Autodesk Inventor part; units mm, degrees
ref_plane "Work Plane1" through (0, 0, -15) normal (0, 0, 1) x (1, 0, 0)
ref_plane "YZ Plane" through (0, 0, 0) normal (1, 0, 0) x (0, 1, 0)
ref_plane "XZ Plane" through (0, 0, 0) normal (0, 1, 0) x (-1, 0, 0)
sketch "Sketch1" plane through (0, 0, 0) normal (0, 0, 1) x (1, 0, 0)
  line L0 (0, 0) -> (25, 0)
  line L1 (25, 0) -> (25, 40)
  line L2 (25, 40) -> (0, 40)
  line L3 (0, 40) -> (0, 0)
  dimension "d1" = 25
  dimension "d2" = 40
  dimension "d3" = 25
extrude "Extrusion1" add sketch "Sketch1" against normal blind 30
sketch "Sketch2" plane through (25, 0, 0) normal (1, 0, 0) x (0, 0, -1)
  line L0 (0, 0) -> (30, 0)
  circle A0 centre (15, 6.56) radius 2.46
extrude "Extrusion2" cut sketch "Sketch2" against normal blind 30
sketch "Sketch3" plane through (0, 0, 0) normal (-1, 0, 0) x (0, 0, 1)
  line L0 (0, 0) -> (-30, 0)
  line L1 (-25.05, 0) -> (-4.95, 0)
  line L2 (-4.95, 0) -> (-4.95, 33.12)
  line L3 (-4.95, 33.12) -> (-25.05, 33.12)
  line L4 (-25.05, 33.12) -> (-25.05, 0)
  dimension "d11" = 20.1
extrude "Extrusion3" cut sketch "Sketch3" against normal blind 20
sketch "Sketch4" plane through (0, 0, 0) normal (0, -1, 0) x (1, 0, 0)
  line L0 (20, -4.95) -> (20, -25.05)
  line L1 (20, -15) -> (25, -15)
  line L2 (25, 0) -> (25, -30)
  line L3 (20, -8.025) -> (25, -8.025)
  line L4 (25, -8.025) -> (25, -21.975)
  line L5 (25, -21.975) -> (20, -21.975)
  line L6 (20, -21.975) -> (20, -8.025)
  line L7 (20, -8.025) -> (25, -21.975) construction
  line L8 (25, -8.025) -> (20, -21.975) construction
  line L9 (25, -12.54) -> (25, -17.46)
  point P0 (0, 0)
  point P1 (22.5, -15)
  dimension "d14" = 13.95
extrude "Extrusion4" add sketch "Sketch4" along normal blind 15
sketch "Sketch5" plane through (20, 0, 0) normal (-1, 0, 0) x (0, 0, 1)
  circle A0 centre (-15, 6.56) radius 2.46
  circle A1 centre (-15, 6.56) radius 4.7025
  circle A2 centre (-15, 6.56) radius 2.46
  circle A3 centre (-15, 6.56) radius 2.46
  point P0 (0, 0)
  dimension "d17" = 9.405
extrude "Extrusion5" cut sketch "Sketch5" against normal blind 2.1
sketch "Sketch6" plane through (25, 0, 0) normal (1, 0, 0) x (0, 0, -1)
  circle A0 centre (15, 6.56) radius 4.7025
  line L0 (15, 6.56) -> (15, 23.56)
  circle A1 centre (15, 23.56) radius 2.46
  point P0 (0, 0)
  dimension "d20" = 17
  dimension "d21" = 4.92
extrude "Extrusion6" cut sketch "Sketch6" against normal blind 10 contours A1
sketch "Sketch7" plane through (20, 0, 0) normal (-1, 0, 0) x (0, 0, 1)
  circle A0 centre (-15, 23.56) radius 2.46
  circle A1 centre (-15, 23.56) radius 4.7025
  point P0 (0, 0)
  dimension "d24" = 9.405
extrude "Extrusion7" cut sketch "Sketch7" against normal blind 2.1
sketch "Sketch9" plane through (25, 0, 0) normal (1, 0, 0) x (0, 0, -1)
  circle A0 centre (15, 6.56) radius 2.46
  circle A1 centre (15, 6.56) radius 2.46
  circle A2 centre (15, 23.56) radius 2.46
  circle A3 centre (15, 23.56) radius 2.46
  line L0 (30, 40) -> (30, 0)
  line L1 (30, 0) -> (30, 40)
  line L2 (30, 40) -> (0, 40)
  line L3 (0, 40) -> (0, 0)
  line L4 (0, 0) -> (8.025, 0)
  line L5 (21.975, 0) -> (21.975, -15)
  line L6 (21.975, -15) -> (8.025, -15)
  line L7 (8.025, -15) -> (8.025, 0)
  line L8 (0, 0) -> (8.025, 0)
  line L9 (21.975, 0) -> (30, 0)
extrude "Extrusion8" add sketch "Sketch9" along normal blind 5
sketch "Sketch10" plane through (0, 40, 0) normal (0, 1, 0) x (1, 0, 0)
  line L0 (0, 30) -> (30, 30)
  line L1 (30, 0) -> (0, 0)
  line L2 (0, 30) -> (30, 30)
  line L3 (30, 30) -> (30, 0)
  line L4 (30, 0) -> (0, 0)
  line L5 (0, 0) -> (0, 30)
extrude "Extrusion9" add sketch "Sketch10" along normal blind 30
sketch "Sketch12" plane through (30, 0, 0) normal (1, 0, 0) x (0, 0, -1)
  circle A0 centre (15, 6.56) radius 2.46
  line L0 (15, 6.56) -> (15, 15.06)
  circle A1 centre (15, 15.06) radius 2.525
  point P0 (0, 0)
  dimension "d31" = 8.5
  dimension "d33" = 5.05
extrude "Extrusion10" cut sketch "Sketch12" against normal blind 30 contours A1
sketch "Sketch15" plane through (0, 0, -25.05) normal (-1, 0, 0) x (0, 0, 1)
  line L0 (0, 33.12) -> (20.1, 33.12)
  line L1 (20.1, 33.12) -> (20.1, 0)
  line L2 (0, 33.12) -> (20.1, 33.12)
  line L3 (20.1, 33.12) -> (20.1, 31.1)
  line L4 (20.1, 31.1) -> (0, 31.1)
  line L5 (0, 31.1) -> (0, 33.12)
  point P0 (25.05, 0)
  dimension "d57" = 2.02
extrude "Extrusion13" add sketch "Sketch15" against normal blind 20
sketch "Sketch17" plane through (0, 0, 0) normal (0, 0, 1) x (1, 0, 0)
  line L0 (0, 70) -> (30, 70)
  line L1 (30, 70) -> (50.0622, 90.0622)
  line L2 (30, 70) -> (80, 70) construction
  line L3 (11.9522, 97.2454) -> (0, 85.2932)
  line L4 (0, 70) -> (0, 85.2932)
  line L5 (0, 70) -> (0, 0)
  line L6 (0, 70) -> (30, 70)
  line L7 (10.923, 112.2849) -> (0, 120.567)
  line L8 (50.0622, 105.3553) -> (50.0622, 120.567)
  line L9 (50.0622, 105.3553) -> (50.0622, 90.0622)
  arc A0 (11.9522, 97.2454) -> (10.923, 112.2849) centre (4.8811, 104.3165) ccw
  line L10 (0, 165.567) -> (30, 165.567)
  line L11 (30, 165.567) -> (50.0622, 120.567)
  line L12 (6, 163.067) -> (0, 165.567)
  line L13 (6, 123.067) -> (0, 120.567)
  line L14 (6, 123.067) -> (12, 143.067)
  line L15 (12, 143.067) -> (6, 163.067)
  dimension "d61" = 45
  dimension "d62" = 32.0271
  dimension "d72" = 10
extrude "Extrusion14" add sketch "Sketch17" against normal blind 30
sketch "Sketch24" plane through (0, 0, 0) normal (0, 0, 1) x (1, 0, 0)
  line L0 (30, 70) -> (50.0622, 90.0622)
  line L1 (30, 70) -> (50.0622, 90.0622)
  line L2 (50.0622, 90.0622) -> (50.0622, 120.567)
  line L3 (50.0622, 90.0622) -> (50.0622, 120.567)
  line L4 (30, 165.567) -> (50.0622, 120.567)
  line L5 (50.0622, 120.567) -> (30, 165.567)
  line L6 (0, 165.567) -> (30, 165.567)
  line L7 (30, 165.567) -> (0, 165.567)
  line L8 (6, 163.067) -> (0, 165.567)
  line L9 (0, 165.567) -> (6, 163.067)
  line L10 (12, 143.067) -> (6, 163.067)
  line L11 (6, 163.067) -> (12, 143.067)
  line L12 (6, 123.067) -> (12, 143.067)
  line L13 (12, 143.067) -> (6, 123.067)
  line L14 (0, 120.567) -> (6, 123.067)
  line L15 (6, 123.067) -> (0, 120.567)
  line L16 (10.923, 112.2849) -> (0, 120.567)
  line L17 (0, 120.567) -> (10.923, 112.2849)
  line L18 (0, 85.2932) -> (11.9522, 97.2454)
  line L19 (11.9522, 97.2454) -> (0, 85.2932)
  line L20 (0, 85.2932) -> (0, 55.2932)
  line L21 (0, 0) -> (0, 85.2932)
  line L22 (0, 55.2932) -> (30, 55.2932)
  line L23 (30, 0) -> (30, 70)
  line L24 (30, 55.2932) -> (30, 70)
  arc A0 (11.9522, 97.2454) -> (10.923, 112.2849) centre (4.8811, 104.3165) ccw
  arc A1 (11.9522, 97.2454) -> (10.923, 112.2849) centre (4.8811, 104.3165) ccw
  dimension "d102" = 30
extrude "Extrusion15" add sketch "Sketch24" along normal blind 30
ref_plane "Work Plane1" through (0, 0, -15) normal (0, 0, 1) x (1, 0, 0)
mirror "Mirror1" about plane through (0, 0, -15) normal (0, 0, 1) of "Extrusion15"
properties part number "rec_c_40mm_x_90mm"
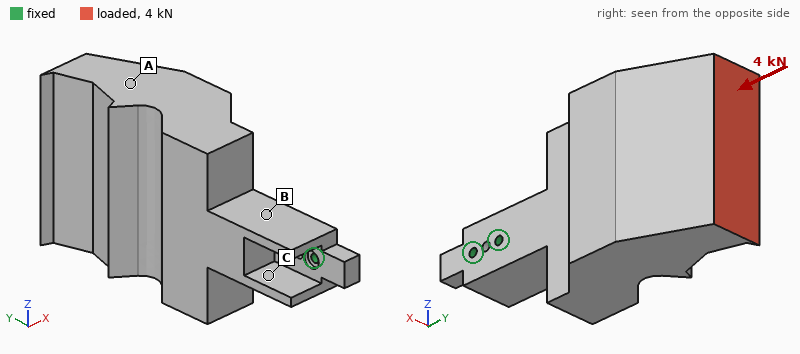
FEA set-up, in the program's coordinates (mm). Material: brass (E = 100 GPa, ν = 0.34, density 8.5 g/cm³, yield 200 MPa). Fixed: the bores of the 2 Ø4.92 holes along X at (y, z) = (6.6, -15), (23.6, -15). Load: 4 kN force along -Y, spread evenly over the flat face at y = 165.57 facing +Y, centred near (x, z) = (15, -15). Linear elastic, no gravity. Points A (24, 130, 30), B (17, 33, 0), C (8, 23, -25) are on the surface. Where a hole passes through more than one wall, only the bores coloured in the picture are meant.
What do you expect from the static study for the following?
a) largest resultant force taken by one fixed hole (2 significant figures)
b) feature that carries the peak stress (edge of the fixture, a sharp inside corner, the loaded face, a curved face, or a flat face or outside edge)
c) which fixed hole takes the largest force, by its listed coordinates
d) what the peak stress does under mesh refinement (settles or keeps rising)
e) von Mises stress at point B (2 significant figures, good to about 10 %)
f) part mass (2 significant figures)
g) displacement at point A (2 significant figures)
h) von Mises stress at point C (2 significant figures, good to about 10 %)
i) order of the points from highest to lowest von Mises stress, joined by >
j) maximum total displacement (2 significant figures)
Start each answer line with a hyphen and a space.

- 3.0 kN
- edge of the fixture
- (23.6, -15)
- keeps rising
- 7.7 MPa
- 3.3 kg
- 0.069 mm
- 13 MPa
- C > B > A
- 0.10 mm
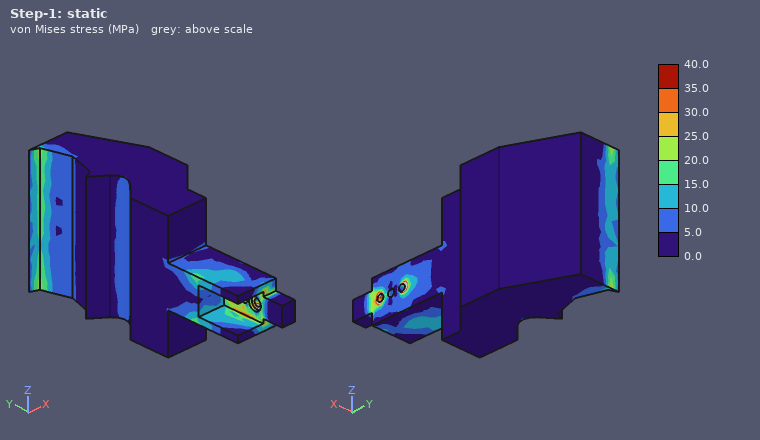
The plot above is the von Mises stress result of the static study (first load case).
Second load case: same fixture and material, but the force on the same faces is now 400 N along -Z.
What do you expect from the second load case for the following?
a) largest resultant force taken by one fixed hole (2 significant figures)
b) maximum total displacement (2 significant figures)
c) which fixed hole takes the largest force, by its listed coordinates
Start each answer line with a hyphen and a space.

- 2.9 kN
- 0.12 mm
- (23.6, -15)
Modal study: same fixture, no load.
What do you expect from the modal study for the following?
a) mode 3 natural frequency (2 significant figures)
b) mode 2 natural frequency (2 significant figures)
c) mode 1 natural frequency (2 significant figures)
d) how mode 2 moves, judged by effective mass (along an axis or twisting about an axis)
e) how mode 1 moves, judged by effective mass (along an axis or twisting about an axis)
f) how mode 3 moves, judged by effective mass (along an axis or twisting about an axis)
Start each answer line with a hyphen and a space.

- 520 Hz
- 260 Hz
- 230 Hz
- along Z
- along X
- twisting about Y
